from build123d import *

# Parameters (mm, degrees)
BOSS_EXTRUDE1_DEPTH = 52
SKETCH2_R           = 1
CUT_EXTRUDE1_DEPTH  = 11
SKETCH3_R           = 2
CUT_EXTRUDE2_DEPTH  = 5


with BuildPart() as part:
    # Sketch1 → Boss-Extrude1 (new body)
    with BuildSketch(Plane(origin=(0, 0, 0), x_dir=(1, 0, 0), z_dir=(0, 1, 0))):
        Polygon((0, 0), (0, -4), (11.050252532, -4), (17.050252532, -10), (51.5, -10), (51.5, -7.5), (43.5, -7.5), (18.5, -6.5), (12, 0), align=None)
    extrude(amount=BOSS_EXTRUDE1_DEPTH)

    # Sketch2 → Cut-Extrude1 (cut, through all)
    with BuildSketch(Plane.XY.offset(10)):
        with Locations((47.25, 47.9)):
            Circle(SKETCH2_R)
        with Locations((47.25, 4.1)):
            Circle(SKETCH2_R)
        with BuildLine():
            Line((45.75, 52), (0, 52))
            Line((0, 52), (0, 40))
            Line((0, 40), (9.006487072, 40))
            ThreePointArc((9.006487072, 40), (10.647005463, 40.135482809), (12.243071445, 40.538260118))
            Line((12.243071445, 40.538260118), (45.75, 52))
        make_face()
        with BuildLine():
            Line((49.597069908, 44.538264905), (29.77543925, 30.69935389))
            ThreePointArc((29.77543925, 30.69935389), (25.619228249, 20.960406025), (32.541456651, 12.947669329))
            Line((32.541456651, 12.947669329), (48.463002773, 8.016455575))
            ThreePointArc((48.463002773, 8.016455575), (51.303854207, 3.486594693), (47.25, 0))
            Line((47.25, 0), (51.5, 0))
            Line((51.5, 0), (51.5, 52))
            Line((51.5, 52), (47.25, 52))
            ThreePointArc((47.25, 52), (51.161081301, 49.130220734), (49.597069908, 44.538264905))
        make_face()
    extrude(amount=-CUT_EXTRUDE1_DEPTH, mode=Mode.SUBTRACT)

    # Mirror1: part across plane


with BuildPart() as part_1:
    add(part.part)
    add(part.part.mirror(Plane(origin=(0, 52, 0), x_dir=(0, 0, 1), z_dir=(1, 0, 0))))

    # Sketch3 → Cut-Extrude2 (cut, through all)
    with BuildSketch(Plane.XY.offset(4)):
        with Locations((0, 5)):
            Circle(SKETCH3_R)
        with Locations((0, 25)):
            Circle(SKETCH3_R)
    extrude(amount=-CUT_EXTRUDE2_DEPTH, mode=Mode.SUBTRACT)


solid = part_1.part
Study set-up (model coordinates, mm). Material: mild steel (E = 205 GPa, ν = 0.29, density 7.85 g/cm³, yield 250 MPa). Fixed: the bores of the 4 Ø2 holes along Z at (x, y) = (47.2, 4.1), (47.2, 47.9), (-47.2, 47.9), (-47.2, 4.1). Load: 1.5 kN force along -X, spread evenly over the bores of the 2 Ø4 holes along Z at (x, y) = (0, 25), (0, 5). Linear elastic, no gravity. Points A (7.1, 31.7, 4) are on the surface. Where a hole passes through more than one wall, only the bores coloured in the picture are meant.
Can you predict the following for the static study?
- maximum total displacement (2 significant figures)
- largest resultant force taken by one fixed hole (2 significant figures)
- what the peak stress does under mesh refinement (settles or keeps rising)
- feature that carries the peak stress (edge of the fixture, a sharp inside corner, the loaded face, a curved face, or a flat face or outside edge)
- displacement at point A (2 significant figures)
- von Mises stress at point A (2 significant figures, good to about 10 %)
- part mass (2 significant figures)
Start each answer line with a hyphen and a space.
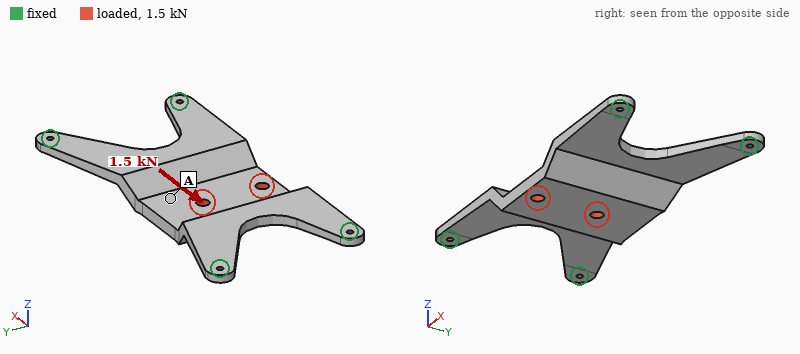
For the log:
- 17 µm
- 450 N
- keeps rising
- edge of the fixture
- 6.6 µm
- 10.0 MPa
- 93 g
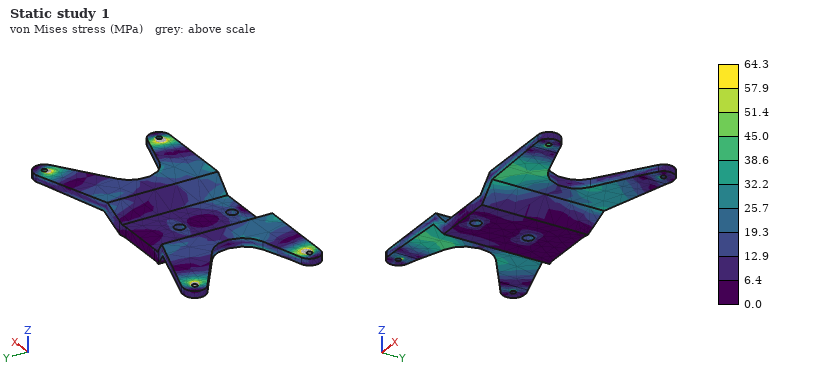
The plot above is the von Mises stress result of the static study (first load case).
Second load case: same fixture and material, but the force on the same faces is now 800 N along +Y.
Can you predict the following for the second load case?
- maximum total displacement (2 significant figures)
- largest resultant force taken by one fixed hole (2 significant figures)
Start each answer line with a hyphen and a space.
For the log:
- 37 µm
- 470 N
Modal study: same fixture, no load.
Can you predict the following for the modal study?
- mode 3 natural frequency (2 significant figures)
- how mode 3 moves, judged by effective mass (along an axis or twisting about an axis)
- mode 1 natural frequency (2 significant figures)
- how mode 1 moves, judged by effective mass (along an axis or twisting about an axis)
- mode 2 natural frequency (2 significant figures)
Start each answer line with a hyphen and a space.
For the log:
- 3600 Hz
- twisting about Y
- 1700 Hz
- along Z
- 2700 Hz
